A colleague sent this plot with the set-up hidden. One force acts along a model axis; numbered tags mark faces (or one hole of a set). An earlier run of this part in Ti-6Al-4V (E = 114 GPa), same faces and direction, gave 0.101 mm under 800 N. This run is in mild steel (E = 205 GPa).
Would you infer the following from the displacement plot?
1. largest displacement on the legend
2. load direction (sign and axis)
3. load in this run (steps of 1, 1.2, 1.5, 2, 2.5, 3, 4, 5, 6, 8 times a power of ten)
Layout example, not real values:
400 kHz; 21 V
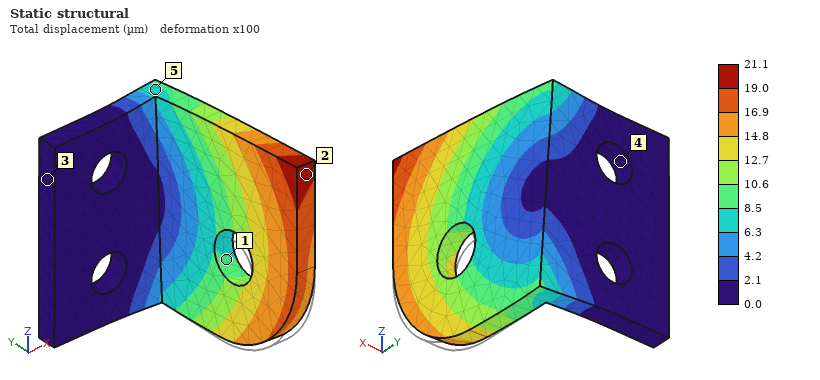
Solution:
21.1 µm; +Z; 300 N
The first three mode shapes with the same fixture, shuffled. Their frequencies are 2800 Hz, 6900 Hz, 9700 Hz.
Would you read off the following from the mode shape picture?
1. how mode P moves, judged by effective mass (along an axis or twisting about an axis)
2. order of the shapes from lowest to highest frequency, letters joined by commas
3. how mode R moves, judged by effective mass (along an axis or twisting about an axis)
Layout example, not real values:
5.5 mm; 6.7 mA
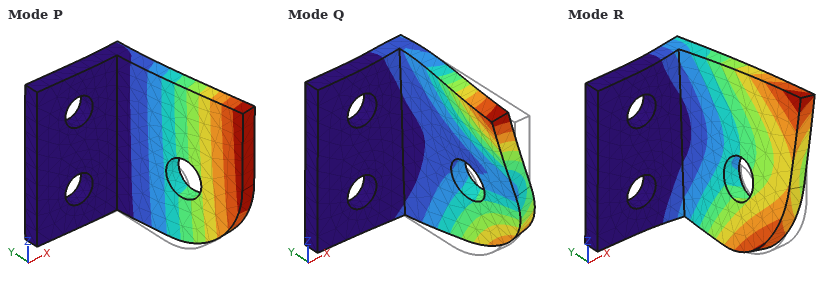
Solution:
along X; P, R, Q; along Z
